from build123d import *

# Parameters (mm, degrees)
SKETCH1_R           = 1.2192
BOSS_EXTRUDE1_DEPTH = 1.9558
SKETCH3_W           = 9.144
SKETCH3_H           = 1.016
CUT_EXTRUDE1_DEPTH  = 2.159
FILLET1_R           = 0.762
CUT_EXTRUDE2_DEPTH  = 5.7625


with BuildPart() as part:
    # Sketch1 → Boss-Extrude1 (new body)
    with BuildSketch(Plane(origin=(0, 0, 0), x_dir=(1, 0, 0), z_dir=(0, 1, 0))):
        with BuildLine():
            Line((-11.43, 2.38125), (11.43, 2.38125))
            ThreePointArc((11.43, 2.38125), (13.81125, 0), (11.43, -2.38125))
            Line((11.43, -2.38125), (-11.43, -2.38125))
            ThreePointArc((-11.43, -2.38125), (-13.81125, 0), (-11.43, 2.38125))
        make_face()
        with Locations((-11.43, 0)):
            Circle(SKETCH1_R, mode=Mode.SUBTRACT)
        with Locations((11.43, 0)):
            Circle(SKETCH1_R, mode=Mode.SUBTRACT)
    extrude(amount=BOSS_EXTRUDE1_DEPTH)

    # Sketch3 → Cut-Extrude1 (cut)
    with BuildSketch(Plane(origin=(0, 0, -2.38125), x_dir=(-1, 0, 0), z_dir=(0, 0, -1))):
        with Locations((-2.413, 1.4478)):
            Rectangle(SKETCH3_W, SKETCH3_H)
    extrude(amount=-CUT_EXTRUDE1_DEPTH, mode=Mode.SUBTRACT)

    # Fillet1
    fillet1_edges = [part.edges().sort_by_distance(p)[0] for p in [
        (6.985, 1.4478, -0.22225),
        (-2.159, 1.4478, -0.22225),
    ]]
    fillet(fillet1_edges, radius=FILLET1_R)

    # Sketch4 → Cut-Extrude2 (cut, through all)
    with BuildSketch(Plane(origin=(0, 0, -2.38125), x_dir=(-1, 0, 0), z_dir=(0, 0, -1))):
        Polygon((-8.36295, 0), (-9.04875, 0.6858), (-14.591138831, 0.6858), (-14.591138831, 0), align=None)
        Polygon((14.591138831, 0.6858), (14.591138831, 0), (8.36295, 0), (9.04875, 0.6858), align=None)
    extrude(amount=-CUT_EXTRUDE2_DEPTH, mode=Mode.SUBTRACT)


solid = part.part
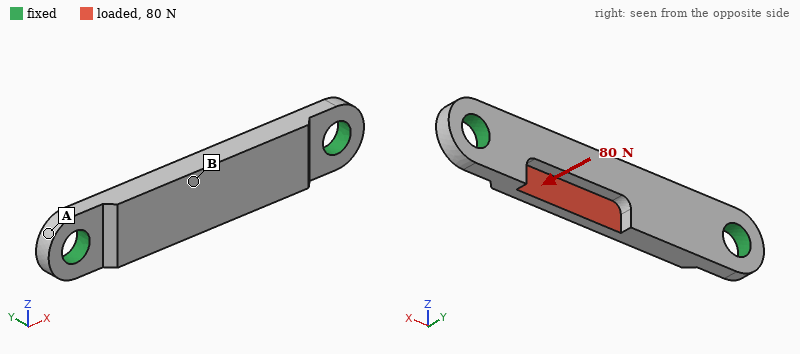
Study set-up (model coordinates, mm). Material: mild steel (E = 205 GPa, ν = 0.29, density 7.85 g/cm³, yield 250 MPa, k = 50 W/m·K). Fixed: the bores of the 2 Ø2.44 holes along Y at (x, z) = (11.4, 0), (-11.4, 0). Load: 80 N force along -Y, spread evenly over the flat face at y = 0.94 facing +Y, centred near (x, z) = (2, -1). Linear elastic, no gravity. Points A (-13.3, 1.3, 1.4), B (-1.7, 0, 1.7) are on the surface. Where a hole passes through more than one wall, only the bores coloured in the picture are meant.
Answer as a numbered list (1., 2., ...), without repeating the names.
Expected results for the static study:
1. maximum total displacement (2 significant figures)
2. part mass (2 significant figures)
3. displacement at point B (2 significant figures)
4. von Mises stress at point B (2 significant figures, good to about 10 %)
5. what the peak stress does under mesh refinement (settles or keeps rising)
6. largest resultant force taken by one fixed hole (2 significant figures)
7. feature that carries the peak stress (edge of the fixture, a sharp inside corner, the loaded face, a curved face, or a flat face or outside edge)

1. 14 µm
2. 1.5 g
3. 7.7 µm
4. 55 MPa
5. keeps rising
6. 96 N
7. edge of the fixture
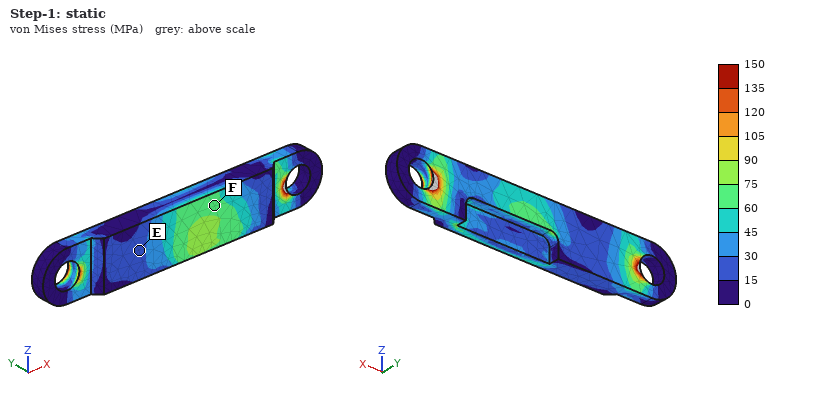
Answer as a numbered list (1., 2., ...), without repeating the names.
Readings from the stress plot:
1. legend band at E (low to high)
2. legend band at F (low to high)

1. 15 to 30 MPa
2. 60 to 75 MPa
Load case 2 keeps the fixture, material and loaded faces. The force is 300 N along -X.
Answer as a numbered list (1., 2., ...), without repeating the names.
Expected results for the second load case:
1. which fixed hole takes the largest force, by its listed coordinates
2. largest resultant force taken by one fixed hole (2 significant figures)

1. (11.4, 0)
2. 170 N
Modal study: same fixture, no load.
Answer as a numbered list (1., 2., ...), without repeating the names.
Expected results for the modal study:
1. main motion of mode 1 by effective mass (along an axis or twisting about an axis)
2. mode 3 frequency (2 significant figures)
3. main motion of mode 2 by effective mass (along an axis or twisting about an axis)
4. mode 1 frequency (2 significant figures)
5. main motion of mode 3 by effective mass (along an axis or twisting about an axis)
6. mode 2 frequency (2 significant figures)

1. along Y
2. 42 kHz
3. along Z
4. 18 kHz
5. twisting about X
6. 35 kHz
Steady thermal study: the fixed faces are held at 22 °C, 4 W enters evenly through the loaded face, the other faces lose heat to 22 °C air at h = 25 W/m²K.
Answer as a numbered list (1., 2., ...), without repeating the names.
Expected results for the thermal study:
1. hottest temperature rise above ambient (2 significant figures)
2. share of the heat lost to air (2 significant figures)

1. 51 K
2. 4.1 %
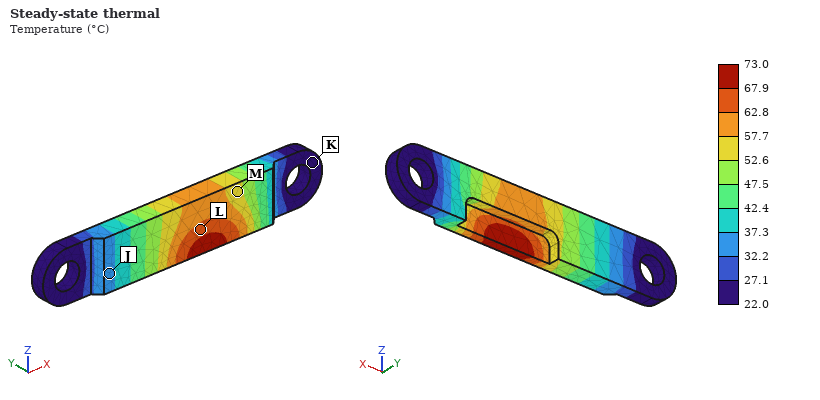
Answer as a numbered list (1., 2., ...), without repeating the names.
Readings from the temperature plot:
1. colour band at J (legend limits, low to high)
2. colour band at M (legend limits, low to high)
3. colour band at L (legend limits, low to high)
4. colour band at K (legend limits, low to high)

1. 32.2 to 37.3 °C
2. 52.6 to 57.7 °C
3. 62.8 to 67.9 °C
4. 22.0 to 27.1 °C
